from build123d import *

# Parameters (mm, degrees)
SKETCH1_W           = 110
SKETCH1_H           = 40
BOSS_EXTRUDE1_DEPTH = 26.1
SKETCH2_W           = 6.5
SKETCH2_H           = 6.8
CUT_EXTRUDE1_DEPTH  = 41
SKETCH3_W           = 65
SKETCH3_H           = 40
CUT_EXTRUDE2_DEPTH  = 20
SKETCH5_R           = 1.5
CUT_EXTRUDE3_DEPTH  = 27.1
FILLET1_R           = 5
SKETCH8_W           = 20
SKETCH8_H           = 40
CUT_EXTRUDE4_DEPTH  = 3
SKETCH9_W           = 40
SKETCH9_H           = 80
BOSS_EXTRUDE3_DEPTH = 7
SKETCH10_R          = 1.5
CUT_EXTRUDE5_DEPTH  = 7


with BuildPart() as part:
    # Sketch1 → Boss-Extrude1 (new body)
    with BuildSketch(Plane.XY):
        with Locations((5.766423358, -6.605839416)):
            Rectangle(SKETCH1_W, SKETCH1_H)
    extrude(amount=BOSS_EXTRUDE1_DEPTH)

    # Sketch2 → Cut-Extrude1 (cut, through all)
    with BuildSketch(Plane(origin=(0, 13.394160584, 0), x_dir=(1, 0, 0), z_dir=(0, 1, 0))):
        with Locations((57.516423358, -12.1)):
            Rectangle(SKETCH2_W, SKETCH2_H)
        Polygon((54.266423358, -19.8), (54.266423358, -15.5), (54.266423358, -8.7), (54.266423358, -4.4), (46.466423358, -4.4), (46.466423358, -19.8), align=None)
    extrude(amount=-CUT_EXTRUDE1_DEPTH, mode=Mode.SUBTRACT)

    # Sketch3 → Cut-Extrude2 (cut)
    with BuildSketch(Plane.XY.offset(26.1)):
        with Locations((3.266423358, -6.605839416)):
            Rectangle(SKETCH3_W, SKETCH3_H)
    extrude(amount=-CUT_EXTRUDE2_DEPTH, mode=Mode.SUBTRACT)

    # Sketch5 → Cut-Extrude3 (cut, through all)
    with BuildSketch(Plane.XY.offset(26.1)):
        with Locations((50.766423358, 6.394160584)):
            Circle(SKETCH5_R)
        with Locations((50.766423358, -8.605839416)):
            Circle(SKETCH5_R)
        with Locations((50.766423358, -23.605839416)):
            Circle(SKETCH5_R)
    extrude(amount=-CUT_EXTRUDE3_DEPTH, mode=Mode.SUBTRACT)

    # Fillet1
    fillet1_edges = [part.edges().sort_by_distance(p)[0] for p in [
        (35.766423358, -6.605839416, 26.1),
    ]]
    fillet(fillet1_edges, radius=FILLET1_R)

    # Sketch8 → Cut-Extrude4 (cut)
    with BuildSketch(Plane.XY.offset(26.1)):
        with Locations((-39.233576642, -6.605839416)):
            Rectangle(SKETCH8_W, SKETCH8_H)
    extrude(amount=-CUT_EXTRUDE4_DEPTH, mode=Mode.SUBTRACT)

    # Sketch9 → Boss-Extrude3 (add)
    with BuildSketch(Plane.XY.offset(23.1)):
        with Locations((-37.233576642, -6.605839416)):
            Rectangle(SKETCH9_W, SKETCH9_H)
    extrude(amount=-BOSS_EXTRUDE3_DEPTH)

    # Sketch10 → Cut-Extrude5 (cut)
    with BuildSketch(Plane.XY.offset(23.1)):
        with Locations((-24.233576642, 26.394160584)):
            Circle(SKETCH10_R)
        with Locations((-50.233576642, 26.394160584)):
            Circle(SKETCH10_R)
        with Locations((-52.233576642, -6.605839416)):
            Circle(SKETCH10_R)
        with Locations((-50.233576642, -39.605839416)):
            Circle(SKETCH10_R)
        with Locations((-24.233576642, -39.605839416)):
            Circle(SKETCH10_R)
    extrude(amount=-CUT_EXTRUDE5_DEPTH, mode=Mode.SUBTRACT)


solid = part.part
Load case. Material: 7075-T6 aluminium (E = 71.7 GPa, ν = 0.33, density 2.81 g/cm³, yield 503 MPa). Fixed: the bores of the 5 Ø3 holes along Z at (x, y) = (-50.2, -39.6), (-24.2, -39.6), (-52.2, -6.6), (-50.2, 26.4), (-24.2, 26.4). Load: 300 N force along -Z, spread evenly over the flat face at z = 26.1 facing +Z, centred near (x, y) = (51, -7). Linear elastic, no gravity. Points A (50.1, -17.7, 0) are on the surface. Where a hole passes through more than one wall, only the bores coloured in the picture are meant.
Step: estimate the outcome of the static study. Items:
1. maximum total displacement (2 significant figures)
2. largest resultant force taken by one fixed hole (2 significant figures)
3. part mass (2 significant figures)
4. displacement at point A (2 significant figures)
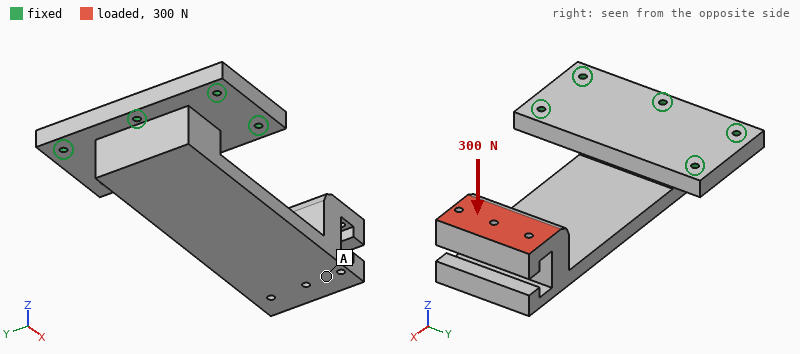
1.4 mm
520 N
200 g
1.1 mm
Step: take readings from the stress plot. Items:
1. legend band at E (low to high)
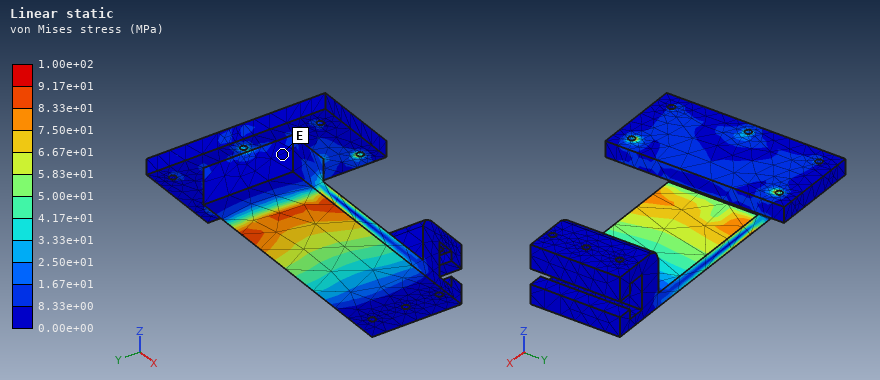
0.00e+00 to 8.33e+00 MPa
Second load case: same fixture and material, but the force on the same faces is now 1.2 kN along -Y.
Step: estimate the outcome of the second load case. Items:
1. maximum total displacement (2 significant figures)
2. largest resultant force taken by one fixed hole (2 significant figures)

0.85 mm
1.0 kN
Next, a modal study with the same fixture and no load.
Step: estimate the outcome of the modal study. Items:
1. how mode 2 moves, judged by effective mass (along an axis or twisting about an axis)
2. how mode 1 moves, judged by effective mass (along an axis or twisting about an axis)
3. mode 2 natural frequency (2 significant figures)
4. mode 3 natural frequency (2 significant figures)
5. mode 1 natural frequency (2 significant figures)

along Y
along Z
1200 Hz
2100 Hz
350 Hz
